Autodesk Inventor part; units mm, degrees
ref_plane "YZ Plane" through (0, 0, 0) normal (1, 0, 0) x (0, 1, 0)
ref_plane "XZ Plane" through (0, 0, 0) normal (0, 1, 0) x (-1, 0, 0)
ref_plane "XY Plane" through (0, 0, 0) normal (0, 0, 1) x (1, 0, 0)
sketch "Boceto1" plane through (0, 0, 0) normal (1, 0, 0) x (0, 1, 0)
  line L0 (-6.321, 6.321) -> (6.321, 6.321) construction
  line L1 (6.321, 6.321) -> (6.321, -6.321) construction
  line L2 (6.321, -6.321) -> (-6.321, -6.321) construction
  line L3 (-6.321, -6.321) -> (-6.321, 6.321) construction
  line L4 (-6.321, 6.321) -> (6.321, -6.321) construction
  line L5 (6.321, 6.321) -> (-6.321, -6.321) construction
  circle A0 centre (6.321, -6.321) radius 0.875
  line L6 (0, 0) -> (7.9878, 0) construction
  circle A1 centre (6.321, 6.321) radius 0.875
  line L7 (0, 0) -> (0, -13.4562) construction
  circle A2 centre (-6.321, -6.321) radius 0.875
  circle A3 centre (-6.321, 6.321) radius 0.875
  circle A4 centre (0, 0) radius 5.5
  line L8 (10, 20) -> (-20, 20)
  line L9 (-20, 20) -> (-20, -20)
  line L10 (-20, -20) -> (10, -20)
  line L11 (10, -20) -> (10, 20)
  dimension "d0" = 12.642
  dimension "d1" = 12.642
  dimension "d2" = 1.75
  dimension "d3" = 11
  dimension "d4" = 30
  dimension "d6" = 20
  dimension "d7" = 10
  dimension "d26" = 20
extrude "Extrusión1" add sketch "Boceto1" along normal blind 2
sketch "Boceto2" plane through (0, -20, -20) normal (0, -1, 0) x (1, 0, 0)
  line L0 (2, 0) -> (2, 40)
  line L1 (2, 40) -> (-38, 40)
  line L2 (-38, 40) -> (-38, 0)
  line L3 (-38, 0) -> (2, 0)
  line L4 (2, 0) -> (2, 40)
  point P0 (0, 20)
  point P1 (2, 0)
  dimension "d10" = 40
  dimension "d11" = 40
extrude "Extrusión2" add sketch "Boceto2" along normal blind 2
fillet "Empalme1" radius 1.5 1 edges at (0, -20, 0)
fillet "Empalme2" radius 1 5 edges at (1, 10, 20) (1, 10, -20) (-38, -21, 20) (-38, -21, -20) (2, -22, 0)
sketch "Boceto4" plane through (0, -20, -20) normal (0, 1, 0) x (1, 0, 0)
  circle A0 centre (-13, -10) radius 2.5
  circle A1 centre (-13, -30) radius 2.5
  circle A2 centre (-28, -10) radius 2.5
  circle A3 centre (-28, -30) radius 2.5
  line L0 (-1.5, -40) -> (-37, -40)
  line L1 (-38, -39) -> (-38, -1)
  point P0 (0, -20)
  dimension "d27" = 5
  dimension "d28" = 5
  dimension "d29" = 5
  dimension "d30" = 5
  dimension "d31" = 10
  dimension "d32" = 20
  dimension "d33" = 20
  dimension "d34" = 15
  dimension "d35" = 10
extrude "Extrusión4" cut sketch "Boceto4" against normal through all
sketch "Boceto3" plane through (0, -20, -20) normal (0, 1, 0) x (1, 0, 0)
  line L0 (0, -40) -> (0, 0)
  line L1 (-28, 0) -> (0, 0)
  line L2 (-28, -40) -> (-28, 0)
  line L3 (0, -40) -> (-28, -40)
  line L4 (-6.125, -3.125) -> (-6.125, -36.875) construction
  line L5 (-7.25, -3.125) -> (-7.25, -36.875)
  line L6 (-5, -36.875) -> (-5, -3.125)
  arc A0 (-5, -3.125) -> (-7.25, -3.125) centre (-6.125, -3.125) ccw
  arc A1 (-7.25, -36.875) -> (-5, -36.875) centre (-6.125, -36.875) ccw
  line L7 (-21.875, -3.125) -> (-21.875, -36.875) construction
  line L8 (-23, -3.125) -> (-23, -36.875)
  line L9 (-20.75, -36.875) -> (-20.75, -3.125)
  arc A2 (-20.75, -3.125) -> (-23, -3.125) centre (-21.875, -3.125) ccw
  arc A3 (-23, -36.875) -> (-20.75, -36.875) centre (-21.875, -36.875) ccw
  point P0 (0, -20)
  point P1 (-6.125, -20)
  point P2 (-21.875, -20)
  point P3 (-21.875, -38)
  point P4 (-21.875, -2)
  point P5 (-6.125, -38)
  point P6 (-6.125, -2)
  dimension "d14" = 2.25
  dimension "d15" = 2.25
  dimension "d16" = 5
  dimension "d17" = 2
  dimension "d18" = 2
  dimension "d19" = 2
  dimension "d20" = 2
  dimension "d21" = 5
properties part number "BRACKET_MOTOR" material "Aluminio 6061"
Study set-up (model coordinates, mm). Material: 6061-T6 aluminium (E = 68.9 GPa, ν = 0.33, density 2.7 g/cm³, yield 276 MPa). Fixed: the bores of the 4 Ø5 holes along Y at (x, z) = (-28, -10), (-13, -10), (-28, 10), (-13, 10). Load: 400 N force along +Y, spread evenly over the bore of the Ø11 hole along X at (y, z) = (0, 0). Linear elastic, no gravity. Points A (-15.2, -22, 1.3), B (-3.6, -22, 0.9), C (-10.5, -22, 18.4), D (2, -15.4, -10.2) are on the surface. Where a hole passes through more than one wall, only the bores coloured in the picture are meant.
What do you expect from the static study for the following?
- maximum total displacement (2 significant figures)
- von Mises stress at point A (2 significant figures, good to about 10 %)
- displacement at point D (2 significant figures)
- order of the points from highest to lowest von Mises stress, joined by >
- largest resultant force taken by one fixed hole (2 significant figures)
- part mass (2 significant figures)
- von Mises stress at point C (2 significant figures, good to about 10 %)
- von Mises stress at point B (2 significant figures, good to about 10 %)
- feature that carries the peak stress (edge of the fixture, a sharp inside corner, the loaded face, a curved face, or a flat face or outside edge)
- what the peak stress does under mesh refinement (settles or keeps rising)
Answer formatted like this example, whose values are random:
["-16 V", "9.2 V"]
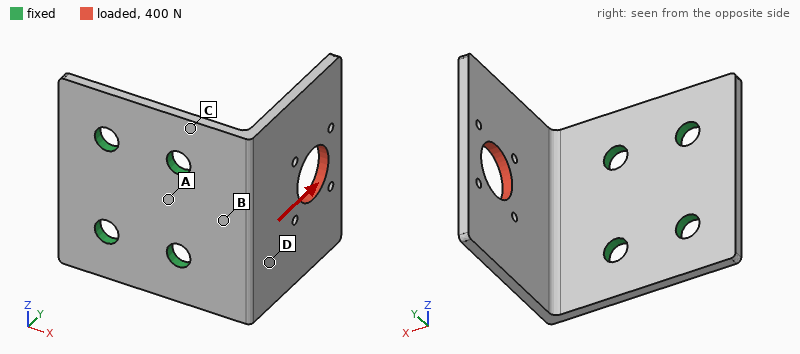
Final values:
["0.55 mm", "33 MPa", "0.19 mm", "C > B > A > D", "220 N", "14 g", "94 MPa", "64 MPa", "edge of the fixture", "keeps rising"]
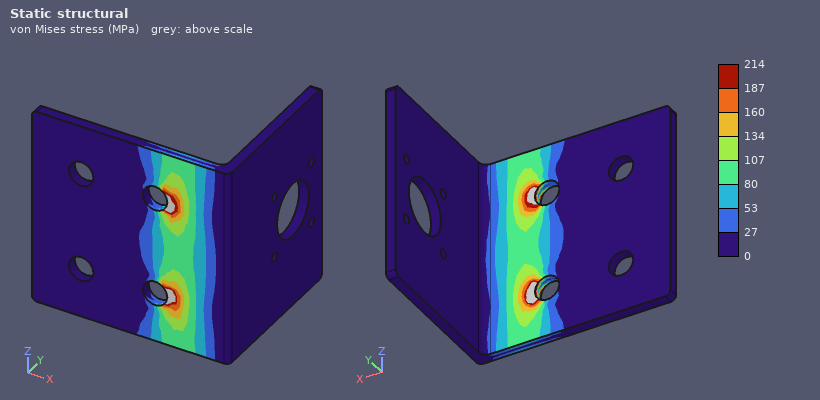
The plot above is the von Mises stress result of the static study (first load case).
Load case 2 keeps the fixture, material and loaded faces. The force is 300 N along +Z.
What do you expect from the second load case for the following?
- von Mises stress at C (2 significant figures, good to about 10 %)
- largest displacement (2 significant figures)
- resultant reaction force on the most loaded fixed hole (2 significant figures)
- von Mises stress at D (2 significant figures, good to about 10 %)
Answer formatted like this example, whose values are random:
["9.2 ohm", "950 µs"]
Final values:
["90 MPa", "0.33 mm", "340 N", "38 MPa"]
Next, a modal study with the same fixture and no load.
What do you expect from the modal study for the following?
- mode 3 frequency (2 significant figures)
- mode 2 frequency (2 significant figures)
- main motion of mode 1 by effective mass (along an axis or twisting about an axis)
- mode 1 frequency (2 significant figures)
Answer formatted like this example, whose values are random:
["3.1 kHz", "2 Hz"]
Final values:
["3500 Hz", "2300 Hz", "along X", "1200 Hz"]
